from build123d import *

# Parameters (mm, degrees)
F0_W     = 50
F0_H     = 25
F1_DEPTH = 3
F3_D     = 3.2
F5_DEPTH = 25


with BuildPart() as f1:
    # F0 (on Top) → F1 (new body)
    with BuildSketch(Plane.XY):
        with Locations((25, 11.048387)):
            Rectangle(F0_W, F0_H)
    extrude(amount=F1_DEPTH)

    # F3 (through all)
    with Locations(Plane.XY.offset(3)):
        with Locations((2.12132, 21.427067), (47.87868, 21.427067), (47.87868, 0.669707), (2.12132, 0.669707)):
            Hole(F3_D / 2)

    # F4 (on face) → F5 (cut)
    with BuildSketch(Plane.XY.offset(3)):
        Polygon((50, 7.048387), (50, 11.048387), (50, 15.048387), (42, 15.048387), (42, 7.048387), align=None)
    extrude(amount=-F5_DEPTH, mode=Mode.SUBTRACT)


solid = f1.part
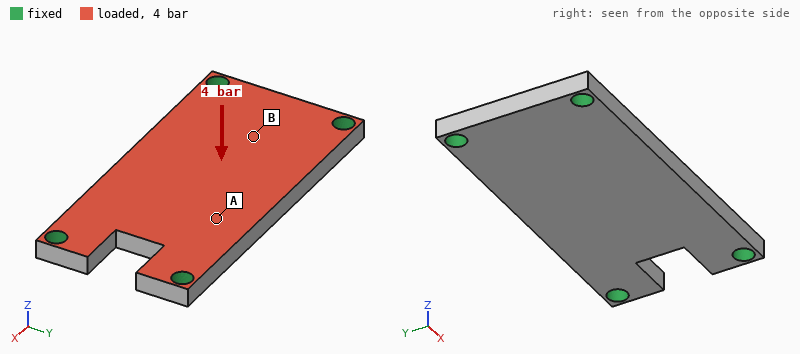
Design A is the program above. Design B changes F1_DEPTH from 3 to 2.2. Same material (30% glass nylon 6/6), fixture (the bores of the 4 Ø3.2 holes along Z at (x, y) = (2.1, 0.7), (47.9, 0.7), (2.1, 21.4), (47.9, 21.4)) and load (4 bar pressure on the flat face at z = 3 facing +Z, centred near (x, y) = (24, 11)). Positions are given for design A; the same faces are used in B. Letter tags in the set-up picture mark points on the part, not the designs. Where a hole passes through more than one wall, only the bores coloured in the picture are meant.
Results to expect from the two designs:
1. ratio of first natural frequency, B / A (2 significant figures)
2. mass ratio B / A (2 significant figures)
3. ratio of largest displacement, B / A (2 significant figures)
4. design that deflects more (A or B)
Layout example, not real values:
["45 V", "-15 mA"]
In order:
["0.76", "0.73", "2.4", "B"]
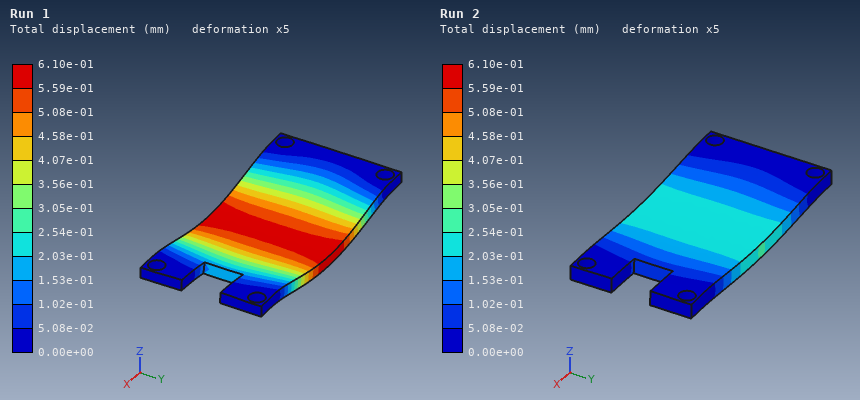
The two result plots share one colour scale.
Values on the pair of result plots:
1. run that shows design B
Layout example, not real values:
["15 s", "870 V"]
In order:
["Run 1"]
